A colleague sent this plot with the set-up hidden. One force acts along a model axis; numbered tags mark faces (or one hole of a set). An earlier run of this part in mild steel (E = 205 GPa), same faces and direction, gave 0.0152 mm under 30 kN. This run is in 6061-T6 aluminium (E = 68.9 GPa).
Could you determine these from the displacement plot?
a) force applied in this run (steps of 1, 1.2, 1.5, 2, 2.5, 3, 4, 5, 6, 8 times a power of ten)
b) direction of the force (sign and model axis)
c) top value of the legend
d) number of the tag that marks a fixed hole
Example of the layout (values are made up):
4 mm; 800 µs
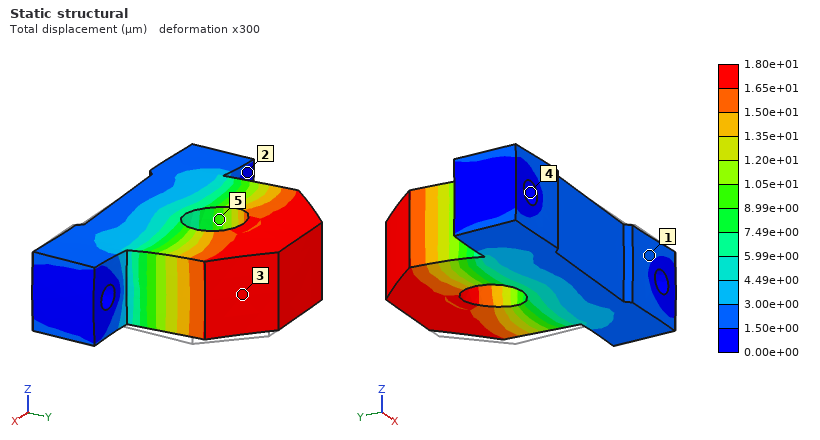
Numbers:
12 kN; -X; 1.80e+01 µm; 4
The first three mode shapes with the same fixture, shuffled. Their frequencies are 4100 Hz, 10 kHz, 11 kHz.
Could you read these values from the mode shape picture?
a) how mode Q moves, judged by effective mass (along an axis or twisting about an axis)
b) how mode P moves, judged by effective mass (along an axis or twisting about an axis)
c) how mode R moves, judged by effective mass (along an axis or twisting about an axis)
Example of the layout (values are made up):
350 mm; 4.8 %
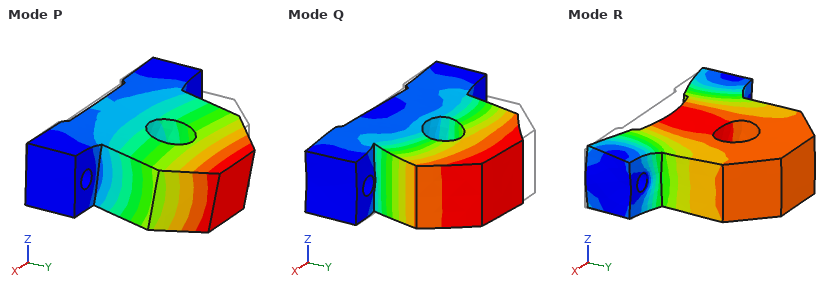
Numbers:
along X; along Z; along Y
